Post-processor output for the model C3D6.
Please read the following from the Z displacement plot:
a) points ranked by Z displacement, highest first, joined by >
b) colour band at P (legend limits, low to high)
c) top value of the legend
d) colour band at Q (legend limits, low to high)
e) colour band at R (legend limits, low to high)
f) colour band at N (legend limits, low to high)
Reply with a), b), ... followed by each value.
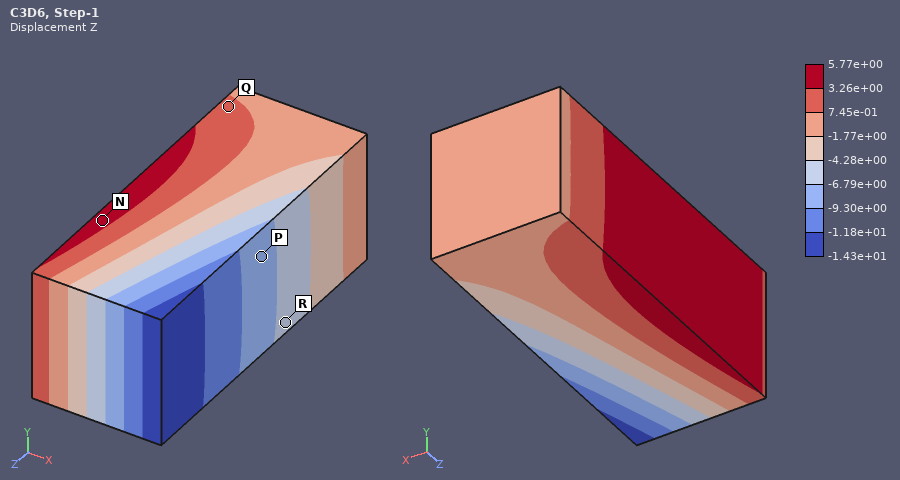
a) N > Q > R > P
b) -9.30e+00 to -6.79e+00
c) 5.77e+00
d) 7.45e-01 to 3.26e+00
e) -6.79e+00 to -4.28e+00
f) 3.26e+00 to 5.77e+00
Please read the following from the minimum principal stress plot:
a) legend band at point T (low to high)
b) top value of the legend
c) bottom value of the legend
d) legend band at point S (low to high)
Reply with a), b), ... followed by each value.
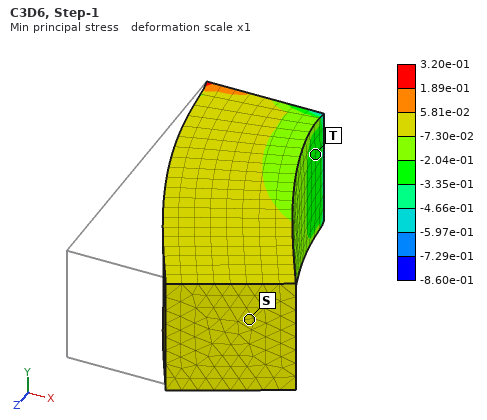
a) -3.35e-01 to -2.04e-01
b) 3.20e-01
c) -8.60e-01
d) -7.30e-02 to 5.81e-02
